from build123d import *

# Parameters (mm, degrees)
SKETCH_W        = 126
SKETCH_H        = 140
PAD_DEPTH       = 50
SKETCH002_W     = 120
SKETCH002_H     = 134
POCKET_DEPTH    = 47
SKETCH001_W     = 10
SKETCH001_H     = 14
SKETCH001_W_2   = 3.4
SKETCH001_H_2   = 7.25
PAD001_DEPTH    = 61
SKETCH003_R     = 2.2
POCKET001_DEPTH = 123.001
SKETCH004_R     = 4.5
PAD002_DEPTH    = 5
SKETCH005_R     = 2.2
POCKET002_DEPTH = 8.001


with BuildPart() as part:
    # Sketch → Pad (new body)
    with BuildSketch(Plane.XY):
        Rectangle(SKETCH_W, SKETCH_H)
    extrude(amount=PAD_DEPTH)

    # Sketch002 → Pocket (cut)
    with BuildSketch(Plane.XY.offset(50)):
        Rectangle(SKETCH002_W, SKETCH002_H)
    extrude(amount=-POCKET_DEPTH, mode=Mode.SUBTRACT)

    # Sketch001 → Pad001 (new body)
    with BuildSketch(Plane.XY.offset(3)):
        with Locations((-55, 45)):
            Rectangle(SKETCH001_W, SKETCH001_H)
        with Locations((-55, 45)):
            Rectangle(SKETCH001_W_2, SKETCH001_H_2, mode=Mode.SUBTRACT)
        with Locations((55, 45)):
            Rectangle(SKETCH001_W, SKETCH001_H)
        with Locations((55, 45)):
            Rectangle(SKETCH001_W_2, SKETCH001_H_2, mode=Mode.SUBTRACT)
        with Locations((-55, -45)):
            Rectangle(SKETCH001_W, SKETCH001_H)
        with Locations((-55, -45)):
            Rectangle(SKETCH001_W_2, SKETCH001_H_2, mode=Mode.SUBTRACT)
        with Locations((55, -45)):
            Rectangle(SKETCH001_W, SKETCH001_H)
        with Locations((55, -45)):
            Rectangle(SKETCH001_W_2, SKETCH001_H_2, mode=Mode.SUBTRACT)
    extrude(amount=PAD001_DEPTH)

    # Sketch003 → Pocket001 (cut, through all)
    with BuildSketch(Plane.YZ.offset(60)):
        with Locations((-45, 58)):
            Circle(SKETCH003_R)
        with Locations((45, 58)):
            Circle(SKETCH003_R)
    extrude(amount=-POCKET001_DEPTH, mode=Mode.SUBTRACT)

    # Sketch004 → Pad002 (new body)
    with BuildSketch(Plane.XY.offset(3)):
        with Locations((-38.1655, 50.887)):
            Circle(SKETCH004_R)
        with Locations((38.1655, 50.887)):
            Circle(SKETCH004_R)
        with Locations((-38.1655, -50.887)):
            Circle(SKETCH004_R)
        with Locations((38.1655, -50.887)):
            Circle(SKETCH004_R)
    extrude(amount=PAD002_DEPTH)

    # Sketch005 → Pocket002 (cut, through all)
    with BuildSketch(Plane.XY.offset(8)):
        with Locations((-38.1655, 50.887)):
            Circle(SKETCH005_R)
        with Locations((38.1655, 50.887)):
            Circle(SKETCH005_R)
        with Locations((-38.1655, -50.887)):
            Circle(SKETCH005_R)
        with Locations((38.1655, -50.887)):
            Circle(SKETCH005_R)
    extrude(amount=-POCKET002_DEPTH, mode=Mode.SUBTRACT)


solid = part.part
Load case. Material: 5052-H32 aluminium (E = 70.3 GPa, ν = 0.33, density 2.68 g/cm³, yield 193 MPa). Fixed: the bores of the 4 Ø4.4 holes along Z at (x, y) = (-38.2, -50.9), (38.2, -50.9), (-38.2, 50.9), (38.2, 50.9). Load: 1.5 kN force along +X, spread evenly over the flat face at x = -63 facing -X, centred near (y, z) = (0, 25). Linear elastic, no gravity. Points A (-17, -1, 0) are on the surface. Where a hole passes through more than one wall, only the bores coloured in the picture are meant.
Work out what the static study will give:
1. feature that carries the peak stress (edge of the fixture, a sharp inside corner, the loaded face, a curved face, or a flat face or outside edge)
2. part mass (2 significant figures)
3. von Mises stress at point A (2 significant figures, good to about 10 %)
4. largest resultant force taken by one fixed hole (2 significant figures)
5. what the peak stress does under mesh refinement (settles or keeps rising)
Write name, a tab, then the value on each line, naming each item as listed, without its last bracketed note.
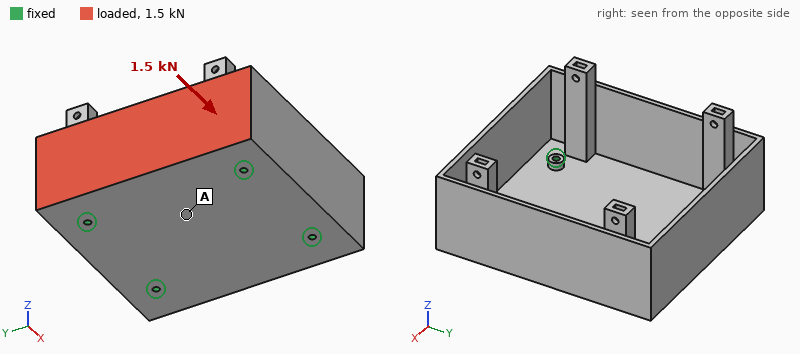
feature that carries the peak stress	edge of the fixture
part mass	410 g
von Mises stress at point A	5.0 MPa
largest resultant force taken by one fixed hole	480 N
what the peak stress does under mesh refinement	keeps rising
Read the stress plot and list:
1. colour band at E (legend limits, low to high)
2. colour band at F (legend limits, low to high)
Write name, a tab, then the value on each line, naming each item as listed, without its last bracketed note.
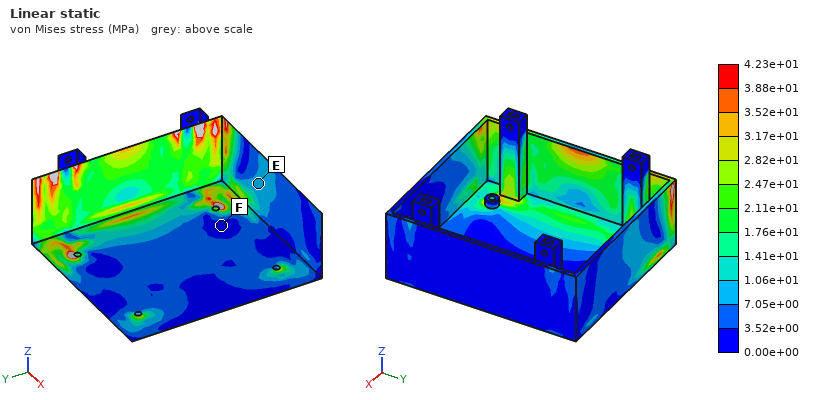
colour band at E	7.05e+00 to 1.06e+01 MPa
colour band at F	0.00e+00 to 3.52e+00 MPa
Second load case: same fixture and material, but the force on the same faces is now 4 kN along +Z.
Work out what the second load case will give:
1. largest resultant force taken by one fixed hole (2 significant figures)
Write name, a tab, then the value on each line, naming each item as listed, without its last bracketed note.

largest resultant force taken by one fixed hole	2.5 kN
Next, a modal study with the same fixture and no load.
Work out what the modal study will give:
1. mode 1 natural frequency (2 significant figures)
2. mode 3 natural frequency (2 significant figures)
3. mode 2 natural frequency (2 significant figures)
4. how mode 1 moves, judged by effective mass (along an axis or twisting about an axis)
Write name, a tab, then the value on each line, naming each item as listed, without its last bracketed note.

mode 1 natural frequency	1300 Hz
mode 3 natural frequency	1400 Hz
mode 2 natural frequency	1400 Hz
how mode 1 moves, judged by effective mass	along X
